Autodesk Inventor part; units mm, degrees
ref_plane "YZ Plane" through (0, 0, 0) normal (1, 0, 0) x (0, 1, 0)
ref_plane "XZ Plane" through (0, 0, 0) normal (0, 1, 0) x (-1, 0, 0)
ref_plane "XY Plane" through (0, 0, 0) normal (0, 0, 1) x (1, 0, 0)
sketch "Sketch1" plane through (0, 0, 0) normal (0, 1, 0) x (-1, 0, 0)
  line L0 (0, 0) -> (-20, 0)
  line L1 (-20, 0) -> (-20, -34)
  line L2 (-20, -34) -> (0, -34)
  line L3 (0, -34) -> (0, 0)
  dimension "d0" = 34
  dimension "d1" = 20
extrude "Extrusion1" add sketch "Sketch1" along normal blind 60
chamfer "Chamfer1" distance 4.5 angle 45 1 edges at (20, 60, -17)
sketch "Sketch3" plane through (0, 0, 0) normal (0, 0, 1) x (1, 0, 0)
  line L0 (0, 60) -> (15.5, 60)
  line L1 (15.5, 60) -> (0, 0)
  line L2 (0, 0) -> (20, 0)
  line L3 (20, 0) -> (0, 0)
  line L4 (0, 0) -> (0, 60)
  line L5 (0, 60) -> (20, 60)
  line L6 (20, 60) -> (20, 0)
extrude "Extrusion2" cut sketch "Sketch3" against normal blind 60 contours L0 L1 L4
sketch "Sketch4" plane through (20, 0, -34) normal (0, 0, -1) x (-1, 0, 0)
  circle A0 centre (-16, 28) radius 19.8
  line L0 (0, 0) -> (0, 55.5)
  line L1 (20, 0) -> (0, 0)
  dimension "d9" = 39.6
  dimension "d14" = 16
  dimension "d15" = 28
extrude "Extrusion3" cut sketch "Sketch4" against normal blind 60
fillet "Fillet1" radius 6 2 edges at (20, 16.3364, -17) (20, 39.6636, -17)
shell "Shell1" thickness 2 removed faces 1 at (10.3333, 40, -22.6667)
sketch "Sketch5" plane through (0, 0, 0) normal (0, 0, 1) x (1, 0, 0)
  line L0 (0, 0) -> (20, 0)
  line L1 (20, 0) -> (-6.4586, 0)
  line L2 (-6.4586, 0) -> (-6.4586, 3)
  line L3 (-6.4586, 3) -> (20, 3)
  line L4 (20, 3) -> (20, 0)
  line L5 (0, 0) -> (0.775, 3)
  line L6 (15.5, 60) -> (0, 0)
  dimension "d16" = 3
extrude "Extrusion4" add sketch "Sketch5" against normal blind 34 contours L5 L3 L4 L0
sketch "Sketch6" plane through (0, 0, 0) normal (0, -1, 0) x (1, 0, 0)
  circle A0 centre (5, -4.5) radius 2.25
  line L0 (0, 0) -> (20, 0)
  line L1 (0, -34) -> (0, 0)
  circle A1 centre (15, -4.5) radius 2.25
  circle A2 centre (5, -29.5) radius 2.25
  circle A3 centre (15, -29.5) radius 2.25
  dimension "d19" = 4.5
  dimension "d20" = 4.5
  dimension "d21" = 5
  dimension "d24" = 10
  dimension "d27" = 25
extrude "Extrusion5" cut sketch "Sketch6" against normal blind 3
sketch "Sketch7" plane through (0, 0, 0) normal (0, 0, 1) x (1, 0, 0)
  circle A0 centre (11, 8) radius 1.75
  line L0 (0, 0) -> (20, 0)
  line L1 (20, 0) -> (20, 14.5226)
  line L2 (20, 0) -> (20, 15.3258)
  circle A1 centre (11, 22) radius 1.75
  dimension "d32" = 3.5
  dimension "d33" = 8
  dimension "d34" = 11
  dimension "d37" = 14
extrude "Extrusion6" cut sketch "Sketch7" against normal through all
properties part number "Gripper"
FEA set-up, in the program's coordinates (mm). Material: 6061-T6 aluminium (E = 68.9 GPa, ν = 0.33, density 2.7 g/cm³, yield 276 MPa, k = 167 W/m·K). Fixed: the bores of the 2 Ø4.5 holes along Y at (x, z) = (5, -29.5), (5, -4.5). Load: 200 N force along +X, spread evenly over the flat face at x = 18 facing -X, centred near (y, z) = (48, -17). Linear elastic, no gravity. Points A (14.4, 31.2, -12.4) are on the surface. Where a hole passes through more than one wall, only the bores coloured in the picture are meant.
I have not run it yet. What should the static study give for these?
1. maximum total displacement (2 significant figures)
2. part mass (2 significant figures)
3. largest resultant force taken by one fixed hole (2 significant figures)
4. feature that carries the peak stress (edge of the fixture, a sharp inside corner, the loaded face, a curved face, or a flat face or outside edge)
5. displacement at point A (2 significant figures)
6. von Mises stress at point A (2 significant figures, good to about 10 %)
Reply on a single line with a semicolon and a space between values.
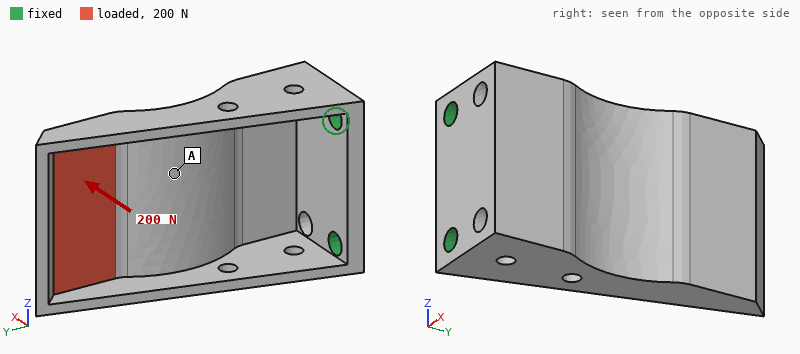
0.34 mm; 21 g; 100 N; edge of the fixture; 0.12 mm; 18 MPa
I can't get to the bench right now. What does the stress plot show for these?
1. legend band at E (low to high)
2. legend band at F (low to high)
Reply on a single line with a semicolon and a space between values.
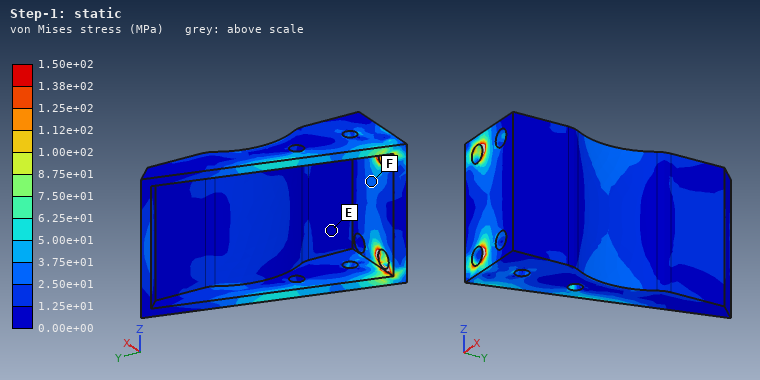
0.00e+00 to 1.25e+01 MPa; 2.50e+01 to 3.75e+01 MPa
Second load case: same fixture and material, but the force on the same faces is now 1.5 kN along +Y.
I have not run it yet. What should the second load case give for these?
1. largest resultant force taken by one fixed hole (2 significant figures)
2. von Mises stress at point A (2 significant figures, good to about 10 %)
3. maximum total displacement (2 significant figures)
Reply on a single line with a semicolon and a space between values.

750 N; 41 MPa; 0.57 mm
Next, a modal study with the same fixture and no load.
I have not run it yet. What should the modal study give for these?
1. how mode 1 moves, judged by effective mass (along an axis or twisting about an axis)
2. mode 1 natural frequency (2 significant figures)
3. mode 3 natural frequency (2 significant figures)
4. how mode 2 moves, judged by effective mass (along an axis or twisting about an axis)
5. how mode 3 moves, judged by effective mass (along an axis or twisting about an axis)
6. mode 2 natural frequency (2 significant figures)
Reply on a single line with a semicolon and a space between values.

along X; 1700 Hz; 6000 Hz; along Z; along Z; 2000 Hz
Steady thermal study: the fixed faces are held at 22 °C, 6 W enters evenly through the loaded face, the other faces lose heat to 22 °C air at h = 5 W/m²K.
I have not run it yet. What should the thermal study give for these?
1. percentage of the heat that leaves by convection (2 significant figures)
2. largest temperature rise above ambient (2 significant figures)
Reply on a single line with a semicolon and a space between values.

5.3 %; 19 K
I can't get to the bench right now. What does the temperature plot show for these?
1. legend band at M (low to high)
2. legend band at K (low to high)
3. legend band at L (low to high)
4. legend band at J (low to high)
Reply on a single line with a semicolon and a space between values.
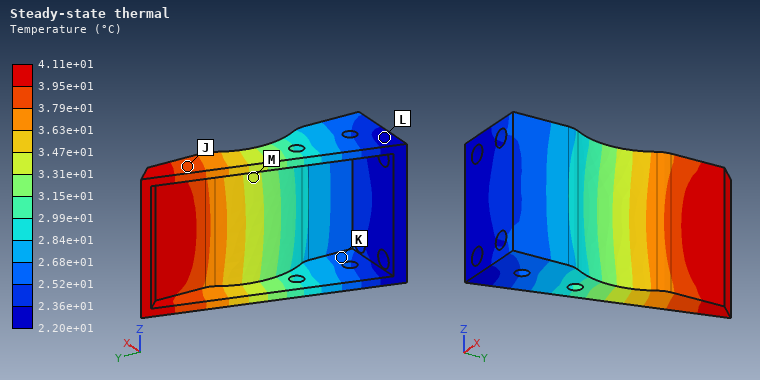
3.31e+01 to 3.47e+01 °C; 2.52e+01 to 2.68e+01 °C; 2.20e+01 to 2.36e+01 °C; 3.79e+01 to 3.95e+01 °C
